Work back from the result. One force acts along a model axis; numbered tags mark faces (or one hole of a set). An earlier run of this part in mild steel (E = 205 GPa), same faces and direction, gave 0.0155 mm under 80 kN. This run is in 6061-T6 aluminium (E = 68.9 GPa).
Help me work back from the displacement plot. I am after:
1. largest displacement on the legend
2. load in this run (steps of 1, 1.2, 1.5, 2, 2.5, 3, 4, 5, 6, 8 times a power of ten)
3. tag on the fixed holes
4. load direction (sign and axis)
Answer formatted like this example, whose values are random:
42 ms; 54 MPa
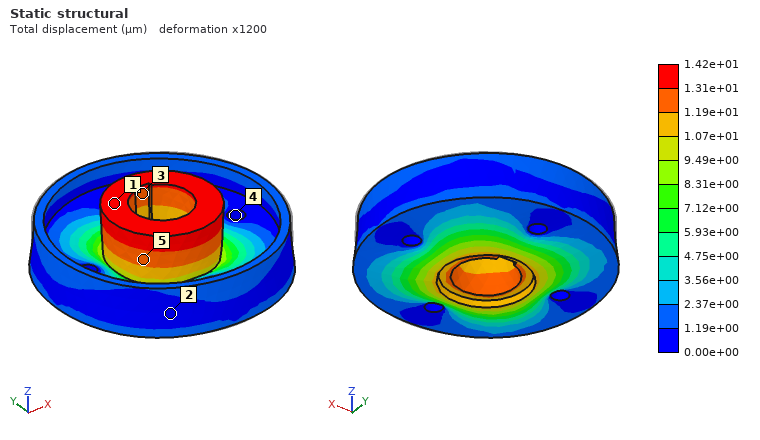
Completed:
1.42e+01 µm; 25 kN; 4; -Z
